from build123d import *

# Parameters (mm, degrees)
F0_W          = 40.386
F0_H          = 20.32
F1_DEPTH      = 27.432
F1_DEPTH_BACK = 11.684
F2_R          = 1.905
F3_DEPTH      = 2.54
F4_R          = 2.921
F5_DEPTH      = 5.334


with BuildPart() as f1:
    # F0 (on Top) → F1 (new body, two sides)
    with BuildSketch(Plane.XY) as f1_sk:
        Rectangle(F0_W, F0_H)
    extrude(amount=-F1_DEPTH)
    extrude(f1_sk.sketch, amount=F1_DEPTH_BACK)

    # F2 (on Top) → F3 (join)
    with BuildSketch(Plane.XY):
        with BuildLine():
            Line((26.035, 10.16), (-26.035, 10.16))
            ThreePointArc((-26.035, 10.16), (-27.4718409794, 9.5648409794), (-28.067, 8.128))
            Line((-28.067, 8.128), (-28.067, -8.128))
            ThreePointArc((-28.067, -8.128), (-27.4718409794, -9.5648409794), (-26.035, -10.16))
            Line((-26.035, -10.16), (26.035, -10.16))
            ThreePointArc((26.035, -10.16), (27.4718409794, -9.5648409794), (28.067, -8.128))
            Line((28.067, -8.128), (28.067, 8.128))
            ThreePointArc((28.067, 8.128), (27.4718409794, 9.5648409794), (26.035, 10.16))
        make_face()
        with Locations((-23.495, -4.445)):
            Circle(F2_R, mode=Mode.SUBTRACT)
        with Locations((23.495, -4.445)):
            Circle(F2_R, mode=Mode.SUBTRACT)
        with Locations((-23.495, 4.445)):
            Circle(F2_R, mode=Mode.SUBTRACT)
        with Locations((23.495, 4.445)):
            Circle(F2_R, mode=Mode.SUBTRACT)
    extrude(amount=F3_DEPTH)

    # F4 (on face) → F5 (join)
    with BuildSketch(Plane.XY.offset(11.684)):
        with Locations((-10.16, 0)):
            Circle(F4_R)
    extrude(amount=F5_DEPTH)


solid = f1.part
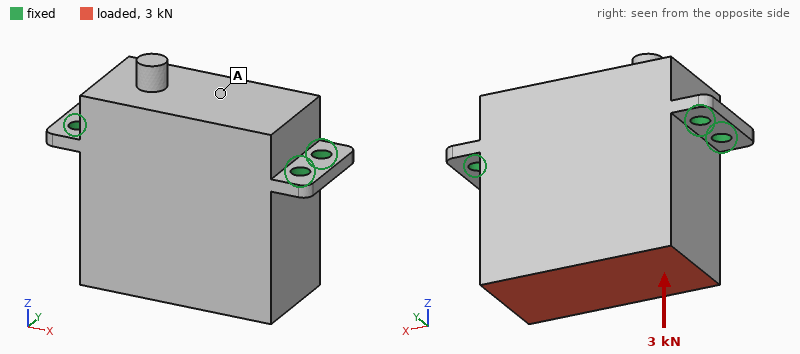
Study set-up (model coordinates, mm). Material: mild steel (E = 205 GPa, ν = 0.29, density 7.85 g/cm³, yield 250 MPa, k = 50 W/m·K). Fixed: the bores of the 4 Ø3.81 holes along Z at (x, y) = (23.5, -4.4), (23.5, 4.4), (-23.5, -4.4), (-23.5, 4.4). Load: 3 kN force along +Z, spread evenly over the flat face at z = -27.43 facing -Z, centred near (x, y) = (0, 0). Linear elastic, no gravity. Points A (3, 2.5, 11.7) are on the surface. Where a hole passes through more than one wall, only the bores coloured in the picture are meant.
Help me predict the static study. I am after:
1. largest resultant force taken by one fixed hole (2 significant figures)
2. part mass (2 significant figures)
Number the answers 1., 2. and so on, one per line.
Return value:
1. 750 N
2. 260 g
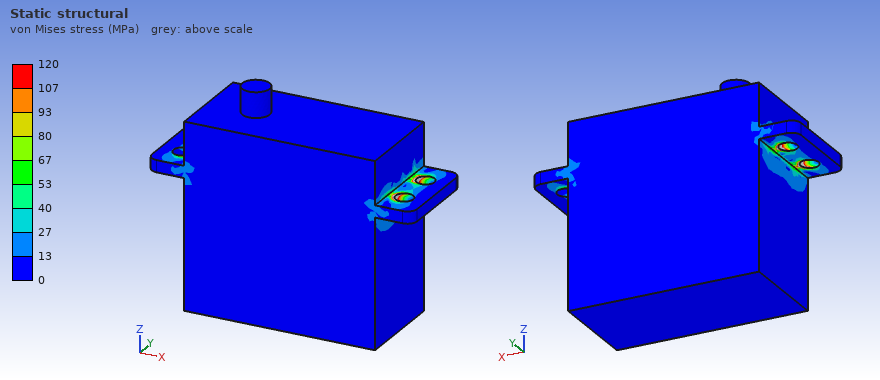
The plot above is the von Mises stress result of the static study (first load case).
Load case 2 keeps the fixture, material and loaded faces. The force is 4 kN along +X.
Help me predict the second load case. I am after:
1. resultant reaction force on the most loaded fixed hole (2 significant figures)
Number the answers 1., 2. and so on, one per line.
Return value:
1. 1.7 kN
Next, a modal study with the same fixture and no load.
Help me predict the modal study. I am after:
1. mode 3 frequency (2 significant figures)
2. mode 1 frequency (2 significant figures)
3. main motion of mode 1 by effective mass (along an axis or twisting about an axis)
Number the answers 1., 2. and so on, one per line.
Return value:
1. 11 kHz
2. 3700 Hz
3. along Y
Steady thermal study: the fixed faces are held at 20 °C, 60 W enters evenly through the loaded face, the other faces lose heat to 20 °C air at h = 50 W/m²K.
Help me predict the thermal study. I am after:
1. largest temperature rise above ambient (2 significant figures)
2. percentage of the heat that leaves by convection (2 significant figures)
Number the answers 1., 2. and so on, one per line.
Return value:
1. 78 K
2. 24 %
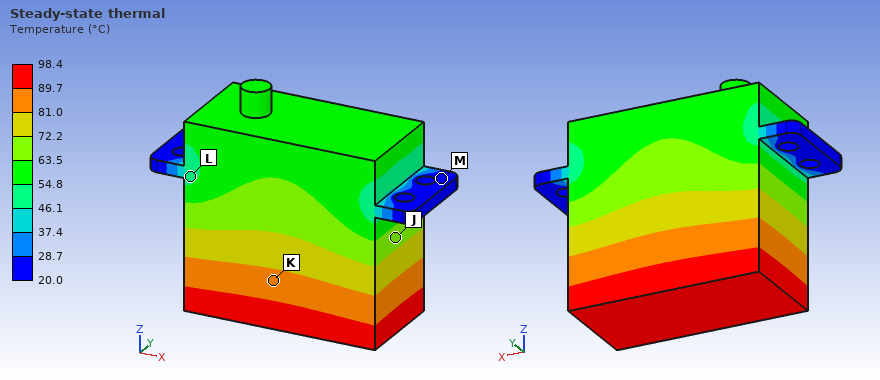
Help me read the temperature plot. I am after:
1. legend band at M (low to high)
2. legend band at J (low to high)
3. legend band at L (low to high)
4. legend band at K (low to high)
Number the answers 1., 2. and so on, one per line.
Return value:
1. 20.0 to 28.7 °C
2. 63.5 to 72.2 °C
3. 46.1 to 54.8 °C
4. 81.0 to 89.7 °C
